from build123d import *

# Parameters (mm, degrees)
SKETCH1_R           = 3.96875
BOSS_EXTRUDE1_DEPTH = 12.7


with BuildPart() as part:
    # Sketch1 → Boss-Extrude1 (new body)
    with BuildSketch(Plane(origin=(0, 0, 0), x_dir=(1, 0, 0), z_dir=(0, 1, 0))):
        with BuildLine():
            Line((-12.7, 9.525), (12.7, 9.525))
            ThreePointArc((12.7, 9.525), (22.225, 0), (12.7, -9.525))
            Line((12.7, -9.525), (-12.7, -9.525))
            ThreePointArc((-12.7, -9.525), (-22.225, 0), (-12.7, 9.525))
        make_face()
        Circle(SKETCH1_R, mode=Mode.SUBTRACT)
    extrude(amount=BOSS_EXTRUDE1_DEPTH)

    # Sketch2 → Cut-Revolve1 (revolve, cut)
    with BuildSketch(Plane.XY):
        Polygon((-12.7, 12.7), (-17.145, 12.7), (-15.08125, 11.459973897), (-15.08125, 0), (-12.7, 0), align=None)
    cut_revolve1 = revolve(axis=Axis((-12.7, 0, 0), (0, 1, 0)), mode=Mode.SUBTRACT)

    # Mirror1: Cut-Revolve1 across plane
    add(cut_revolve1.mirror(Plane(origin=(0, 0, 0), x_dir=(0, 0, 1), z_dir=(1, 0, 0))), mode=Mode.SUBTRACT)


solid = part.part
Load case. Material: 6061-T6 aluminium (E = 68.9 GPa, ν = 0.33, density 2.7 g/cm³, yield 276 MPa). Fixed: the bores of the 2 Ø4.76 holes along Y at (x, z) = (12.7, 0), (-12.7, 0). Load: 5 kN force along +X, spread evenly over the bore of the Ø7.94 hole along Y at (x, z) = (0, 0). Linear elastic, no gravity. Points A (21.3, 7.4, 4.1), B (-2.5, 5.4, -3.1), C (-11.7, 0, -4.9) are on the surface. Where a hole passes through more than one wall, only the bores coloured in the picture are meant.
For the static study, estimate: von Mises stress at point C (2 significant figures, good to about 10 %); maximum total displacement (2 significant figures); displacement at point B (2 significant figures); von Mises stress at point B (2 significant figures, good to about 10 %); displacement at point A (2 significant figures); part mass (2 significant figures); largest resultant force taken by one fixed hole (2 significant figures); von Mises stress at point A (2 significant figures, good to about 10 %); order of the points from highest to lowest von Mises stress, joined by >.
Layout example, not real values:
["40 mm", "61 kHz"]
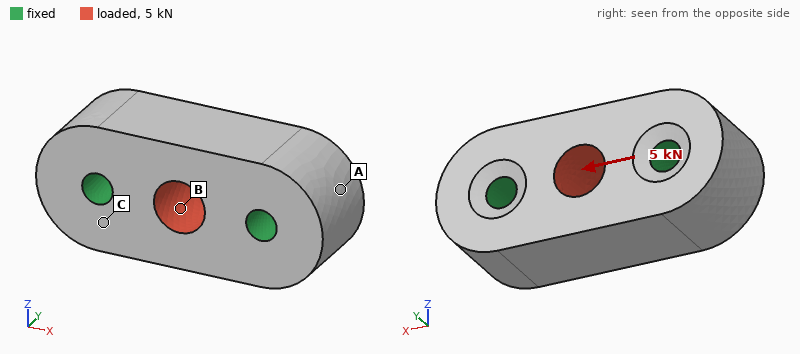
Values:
["7.3 MPa", "2.8 µm", "2.5 µm", "23 MPa", "0.50 µm", "23 g", "2.5 kN", "3.5 MPa", "B > C > A"]
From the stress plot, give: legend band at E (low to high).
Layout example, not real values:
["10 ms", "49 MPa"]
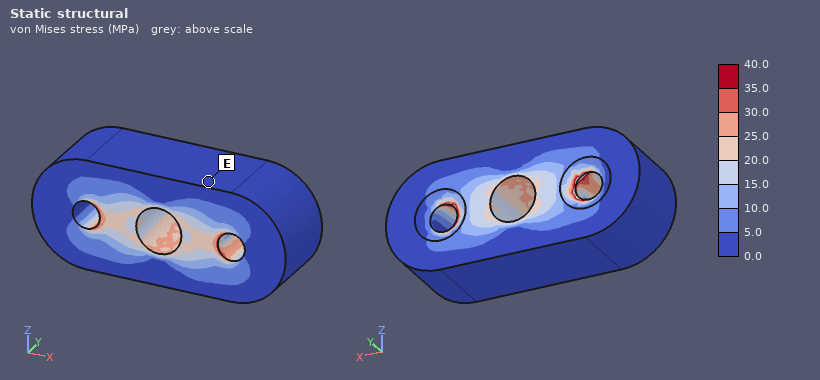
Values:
["0.0 to 5.0 MPa"]
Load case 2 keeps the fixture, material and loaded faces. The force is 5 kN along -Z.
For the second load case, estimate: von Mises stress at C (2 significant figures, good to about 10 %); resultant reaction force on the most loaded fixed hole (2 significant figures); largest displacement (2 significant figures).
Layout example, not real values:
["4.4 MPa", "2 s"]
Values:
["7.2 MPa", "2.5 kN", "7.3 µm"]
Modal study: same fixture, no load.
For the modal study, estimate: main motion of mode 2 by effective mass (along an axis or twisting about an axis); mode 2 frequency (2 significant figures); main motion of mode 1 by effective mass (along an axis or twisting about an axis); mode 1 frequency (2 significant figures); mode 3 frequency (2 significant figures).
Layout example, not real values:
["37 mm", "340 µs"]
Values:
["along Y", "46 kHz", "twisting about X", "44 kHz", "51 kHz"]
